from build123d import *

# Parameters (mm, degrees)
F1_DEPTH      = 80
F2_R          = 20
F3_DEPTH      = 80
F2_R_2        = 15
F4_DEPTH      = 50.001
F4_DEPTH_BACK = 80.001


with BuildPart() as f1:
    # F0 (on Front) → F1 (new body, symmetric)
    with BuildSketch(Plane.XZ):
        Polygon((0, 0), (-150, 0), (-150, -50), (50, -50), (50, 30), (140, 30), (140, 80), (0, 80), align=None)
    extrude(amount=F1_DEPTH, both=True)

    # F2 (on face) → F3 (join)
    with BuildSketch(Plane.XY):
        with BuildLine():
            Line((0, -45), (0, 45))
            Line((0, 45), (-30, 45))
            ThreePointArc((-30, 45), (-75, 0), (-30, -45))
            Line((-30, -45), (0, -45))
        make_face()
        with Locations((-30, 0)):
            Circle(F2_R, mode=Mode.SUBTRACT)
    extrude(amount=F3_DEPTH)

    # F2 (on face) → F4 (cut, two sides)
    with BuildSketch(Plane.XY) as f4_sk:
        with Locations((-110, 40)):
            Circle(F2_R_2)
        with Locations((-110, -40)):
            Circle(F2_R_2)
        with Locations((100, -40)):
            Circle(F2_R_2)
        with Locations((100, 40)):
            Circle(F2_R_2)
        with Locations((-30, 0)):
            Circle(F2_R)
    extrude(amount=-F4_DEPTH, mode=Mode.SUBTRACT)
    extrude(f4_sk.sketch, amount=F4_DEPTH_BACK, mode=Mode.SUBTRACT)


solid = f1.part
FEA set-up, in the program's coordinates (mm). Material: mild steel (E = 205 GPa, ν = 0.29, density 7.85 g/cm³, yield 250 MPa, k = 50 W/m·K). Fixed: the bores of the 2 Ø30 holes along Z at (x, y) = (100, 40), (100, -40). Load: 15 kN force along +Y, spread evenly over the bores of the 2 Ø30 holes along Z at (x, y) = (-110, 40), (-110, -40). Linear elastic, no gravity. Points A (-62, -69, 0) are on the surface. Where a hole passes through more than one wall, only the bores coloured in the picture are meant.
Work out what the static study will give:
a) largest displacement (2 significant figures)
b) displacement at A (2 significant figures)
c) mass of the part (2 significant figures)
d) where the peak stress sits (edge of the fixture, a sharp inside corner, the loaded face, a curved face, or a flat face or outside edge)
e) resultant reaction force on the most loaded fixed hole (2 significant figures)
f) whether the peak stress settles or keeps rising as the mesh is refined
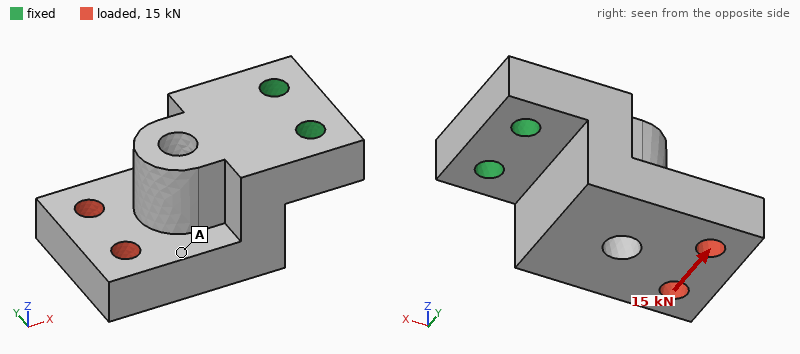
39 µm
23 µm
25 kg
edge of the fixture
33 kN
keeps rising
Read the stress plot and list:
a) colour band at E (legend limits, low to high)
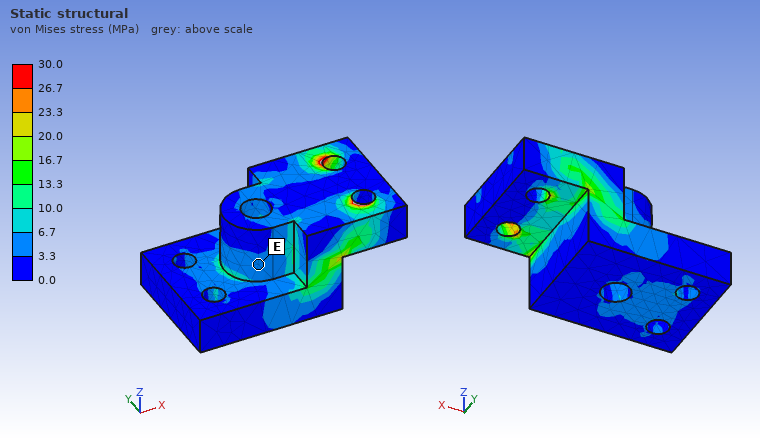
3.3 to 6.7 MPa
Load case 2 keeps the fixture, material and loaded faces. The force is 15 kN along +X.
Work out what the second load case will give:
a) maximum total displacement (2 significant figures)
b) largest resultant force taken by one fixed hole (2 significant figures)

61 µm
7.6 kN
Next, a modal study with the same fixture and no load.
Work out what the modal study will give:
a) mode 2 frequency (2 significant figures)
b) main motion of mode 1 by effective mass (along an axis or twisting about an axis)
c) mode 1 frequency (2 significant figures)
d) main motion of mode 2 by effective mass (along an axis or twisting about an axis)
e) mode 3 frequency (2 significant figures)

1300 Hz
along Z
620 Hz
along Y
2100 Hz
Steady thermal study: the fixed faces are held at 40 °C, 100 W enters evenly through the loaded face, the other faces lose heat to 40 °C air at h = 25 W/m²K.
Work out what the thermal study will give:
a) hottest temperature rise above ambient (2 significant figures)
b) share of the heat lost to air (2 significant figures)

33 K
59 %
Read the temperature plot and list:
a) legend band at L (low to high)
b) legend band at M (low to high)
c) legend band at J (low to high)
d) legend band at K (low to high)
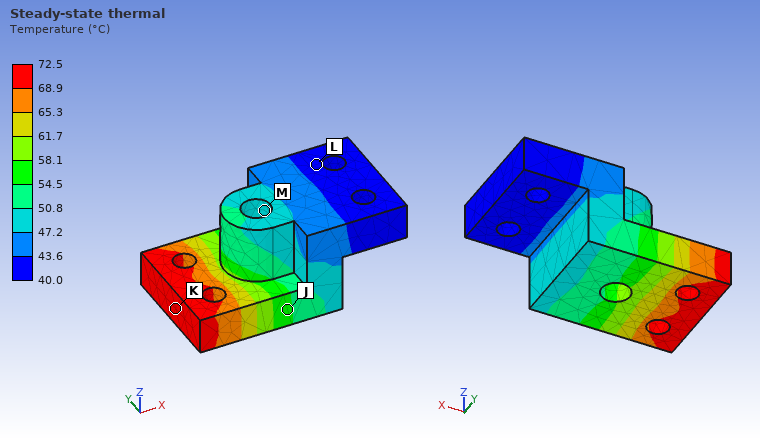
40.0 to 43.6 °C
47.2 to 50.8 °C
54.5 to 58.1 °C
68.9 to 72.5 °C
